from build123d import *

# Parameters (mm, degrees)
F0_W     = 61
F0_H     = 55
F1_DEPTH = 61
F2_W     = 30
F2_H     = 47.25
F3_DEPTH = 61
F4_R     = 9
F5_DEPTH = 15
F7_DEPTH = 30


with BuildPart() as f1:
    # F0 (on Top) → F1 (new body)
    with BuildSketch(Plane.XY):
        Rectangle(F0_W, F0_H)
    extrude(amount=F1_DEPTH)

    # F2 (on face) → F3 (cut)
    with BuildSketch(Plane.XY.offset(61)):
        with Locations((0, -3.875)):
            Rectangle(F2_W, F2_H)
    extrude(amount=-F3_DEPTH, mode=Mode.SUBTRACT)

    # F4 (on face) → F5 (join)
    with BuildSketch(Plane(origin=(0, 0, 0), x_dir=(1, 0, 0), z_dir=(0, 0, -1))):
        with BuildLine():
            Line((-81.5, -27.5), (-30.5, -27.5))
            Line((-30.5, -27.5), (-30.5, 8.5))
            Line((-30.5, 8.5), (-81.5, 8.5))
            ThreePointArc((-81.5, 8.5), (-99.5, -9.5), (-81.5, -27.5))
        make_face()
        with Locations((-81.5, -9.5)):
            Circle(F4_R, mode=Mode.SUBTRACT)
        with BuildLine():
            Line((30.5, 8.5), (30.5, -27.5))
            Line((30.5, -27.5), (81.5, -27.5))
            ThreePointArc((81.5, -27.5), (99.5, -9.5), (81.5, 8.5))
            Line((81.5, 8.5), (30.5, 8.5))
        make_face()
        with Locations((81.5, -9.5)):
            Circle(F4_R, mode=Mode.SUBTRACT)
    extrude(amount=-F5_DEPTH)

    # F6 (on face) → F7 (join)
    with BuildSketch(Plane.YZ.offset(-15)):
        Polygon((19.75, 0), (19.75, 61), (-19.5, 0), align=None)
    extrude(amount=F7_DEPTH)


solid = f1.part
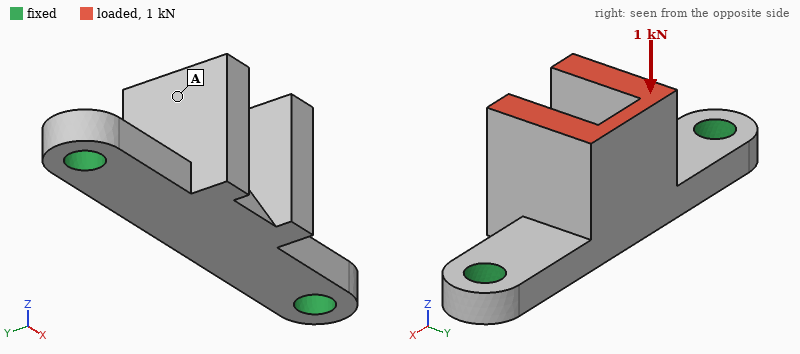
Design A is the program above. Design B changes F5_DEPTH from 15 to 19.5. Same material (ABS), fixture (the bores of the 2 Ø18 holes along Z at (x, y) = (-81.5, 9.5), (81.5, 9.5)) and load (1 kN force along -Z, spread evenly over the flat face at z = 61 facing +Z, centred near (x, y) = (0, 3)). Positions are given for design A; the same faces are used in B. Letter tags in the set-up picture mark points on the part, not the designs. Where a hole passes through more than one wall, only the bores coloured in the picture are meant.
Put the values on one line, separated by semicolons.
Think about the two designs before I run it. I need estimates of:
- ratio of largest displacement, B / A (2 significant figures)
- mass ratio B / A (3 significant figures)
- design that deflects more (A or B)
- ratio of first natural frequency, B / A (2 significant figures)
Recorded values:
0.57; 1.09; A; 1.4
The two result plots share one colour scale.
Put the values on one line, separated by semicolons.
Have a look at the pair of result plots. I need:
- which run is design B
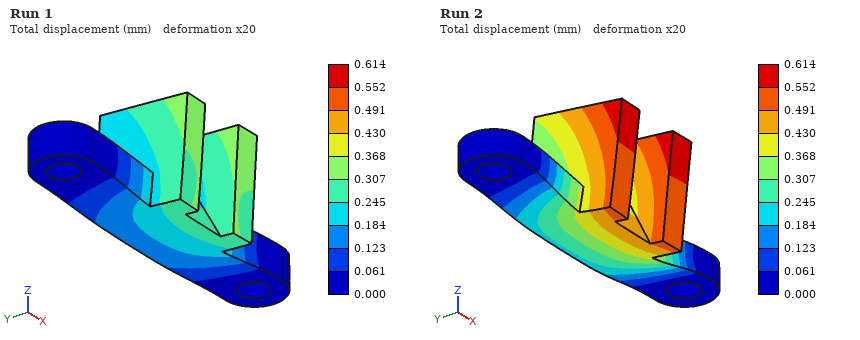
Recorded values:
Run 1
